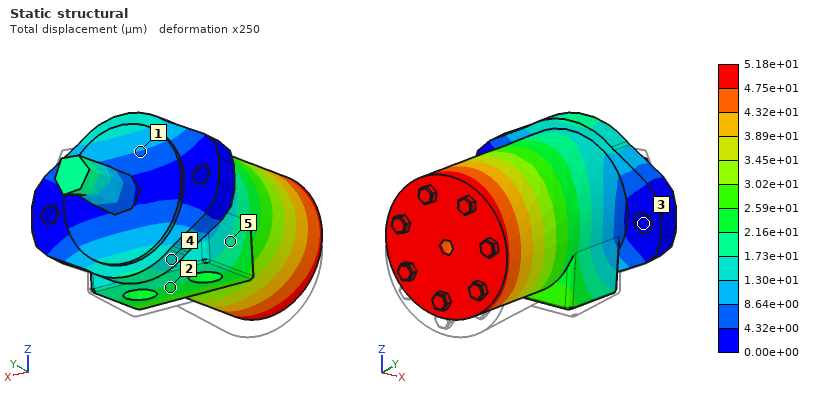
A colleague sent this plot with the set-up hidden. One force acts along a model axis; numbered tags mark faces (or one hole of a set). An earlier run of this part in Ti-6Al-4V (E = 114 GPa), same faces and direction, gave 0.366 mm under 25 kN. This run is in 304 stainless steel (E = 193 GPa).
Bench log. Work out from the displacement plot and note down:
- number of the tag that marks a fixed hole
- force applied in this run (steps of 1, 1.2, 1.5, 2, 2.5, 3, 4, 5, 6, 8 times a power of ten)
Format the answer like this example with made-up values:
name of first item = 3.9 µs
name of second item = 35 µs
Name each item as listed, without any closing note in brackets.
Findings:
number of the tag that marks a fixed hole = 3
force applied in this run = 6 kN
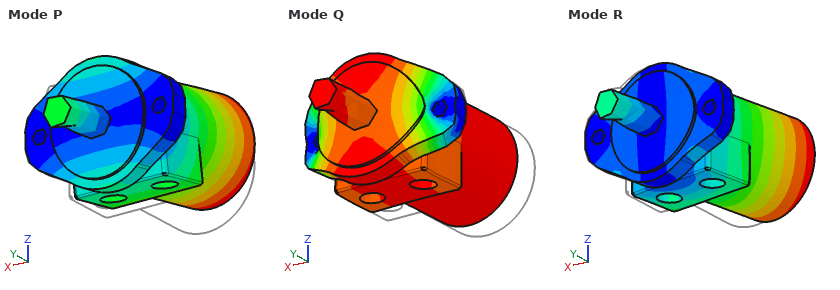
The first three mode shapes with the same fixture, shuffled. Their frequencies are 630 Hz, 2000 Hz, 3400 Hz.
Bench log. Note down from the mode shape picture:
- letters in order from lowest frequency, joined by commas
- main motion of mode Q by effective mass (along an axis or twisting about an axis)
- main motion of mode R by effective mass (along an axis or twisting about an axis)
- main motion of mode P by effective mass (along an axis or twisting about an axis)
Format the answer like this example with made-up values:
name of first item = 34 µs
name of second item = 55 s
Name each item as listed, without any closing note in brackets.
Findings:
letters in order from lowest frequency, joined by commas = P, R, Q
main motion of mode Q by effective mass = along Y
main motion of mode R by effective mass = along X
main motion of mode P by effective mass = along Z
